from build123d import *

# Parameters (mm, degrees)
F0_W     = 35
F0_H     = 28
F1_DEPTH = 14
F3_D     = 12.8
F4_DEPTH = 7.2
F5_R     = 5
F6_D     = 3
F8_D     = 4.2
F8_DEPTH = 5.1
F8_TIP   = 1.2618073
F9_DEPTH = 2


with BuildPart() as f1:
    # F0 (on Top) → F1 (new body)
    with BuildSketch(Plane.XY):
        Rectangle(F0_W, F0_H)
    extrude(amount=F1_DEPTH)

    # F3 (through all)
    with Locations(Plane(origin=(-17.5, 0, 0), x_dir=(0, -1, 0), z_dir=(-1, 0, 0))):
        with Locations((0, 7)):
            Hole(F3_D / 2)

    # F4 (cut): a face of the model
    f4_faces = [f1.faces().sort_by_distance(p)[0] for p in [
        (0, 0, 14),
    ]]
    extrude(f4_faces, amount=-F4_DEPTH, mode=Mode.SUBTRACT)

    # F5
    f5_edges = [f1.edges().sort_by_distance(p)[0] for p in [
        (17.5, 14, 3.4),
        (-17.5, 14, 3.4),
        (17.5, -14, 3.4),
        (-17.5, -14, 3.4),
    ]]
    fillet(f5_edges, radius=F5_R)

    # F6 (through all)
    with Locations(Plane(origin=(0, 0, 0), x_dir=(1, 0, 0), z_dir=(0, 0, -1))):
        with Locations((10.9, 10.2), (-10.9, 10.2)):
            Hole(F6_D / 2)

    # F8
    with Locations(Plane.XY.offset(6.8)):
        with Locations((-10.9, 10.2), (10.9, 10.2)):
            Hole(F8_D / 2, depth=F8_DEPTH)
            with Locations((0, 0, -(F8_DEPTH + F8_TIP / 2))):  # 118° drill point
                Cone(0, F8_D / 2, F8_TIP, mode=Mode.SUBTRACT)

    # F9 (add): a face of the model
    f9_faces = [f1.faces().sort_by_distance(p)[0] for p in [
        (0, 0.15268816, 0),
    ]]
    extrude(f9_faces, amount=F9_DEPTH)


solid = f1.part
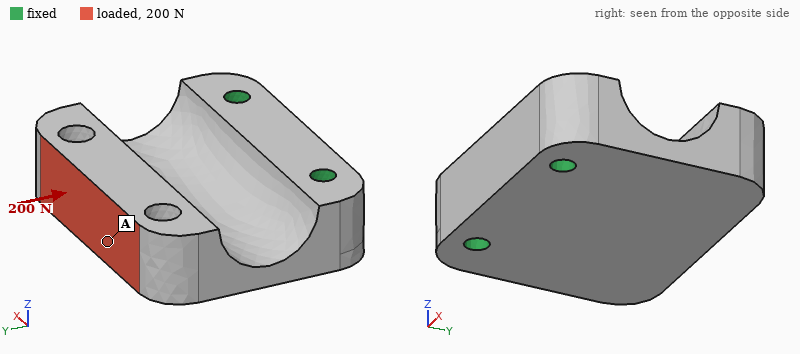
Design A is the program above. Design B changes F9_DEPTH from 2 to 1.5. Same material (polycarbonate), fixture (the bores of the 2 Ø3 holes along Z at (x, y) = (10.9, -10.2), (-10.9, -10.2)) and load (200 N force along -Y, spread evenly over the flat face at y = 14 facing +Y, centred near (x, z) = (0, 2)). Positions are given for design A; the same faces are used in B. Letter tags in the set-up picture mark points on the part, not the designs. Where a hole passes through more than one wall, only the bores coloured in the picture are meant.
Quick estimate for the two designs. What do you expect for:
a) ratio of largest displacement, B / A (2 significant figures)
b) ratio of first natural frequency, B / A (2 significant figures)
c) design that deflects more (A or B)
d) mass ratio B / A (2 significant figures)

1.7
0.81
B
0.92
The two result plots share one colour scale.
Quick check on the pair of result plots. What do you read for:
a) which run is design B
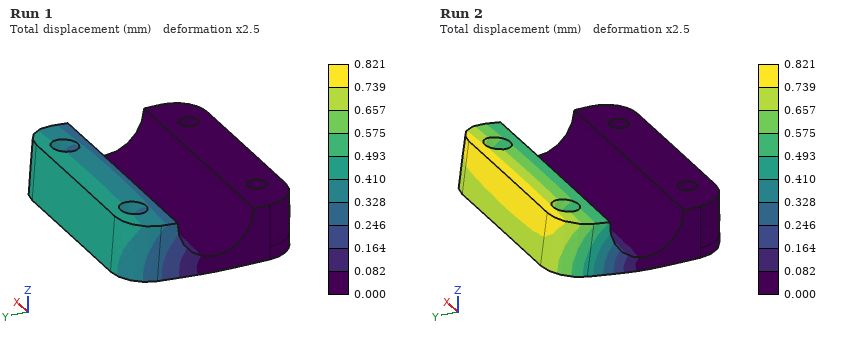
Run 2
